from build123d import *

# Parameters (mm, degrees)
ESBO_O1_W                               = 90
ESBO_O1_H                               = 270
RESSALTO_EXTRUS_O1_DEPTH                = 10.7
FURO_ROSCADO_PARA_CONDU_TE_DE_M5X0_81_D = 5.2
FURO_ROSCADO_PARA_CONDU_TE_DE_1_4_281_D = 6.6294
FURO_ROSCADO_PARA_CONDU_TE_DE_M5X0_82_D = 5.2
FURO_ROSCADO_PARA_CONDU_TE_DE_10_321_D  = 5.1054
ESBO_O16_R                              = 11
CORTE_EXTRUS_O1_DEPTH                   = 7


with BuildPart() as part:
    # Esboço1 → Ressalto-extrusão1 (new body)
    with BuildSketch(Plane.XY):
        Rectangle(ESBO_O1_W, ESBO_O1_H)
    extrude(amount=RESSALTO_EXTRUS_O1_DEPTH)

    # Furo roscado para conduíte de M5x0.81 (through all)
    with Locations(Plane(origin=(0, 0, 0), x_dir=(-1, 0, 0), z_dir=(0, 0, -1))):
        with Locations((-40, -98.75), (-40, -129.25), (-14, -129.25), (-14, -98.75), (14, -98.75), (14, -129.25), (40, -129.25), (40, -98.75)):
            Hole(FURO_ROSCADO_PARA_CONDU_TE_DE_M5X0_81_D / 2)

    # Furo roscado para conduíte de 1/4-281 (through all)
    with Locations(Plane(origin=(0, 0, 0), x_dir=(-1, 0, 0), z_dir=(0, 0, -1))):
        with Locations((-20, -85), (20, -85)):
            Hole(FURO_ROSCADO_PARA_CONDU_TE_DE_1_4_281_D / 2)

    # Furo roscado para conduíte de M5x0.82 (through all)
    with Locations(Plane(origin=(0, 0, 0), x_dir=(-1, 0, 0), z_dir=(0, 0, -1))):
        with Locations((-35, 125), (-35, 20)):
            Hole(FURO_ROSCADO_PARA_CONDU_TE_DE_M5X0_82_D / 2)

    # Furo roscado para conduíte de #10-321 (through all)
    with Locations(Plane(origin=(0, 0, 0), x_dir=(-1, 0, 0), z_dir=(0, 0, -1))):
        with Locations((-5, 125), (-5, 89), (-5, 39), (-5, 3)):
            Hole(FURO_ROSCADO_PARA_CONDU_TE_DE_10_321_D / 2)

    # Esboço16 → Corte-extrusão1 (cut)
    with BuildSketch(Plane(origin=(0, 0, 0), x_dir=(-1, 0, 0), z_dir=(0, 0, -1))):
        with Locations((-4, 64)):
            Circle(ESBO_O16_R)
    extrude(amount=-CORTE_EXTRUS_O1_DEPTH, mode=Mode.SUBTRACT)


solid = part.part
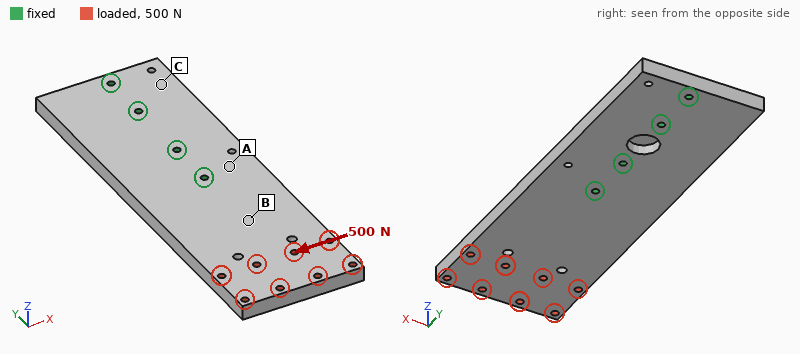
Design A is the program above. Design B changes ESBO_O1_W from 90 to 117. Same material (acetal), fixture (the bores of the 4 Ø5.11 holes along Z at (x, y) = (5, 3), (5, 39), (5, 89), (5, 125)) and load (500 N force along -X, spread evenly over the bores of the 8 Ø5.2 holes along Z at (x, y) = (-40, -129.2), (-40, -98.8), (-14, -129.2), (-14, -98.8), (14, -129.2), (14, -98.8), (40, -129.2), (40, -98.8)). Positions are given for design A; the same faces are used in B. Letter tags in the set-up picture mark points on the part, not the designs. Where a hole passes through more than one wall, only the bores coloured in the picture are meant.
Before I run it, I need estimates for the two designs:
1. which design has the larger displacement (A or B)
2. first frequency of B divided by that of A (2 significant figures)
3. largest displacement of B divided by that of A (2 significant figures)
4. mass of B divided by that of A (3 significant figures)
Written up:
A
0.97
0.61
1.31
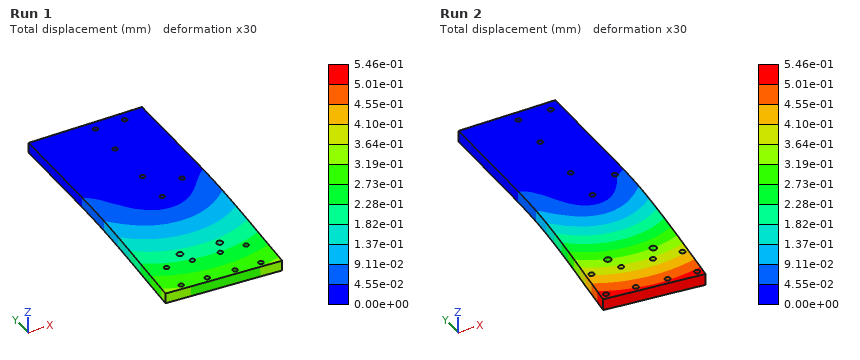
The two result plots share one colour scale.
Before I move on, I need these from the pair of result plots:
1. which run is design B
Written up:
Run 1
